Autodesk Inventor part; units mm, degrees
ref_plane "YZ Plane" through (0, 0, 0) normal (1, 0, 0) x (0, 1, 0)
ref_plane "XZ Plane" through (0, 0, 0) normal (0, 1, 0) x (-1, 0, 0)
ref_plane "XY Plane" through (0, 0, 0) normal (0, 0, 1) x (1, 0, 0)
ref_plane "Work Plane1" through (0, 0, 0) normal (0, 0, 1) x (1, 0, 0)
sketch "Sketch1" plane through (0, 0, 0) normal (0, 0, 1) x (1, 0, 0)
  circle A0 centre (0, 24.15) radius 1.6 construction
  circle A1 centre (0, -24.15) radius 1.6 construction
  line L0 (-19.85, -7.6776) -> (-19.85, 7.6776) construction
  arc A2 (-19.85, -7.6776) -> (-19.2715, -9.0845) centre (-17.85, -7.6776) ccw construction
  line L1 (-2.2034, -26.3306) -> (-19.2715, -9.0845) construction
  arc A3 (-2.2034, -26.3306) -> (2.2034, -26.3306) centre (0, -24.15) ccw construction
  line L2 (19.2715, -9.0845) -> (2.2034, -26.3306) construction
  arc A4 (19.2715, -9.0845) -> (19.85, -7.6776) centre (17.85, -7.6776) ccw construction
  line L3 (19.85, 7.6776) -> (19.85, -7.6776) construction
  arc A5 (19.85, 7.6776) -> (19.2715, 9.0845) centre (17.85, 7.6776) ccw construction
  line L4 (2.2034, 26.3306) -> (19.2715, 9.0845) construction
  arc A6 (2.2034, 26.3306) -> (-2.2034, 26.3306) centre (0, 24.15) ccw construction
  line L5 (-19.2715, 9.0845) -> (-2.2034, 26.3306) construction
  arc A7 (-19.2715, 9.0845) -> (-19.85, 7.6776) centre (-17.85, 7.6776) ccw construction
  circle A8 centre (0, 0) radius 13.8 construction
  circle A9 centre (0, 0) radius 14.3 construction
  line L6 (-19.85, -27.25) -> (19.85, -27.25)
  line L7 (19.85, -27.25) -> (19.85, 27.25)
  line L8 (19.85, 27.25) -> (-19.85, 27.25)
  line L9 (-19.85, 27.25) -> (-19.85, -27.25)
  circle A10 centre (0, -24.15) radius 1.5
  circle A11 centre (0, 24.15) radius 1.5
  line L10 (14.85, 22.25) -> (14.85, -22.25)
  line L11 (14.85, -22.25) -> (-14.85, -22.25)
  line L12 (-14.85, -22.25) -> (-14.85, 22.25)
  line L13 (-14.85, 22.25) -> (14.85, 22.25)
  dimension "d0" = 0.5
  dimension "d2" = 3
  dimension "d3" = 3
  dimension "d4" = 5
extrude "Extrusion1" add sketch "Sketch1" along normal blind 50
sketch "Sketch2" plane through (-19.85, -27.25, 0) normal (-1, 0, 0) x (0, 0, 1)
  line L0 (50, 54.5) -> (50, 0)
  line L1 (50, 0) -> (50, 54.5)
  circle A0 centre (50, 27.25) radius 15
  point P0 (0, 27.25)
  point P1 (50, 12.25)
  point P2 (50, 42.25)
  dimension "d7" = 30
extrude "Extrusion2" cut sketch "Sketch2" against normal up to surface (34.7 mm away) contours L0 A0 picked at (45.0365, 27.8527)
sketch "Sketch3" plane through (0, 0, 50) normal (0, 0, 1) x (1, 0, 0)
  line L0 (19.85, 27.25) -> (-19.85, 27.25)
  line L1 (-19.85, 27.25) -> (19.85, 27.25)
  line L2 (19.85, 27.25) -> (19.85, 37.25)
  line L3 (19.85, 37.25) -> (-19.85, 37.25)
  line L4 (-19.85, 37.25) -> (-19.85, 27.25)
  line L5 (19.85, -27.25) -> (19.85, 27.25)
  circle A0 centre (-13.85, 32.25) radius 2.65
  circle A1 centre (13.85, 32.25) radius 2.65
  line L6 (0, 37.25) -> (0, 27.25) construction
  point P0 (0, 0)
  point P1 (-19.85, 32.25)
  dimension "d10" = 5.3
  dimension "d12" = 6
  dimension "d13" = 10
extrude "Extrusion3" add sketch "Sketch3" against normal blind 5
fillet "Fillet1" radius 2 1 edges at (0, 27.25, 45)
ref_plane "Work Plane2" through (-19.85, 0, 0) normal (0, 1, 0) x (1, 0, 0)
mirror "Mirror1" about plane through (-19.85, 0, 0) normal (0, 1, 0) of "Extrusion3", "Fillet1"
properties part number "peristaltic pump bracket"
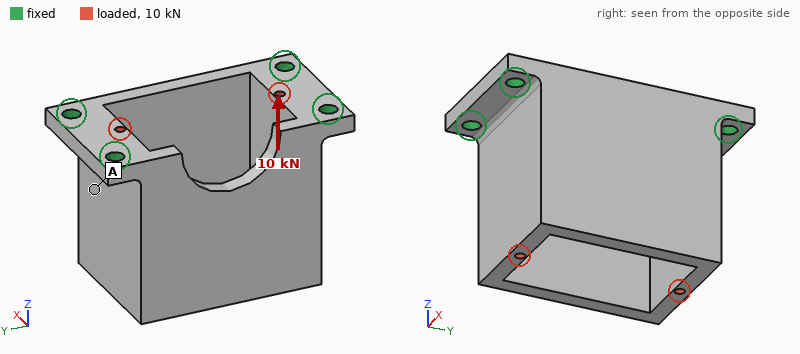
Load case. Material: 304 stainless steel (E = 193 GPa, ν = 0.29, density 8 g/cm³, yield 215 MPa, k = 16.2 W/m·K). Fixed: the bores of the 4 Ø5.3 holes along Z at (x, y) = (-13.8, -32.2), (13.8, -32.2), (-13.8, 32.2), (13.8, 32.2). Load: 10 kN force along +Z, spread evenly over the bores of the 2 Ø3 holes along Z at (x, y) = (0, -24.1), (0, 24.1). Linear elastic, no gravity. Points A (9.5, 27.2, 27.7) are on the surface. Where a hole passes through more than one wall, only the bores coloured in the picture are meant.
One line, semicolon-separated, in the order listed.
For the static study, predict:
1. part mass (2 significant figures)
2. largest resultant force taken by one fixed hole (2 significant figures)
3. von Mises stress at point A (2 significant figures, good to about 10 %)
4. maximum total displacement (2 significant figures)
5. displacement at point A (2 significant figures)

350 g; 2.6 kN; 22 MPa; 9.9 µm; 7.6 µm
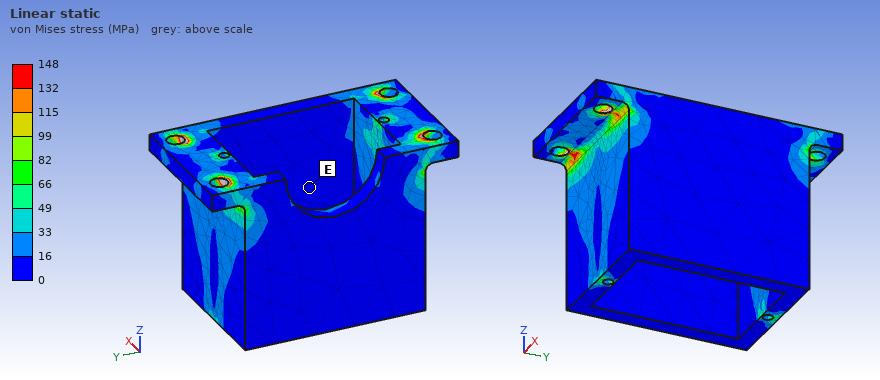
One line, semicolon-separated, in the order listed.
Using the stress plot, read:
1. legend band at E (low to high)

0 to 16 MPa
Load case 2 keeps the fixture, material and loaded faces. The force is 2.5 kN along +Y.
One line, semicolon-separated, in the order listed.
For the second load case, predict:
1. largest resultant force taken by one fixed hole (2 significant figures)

790 N
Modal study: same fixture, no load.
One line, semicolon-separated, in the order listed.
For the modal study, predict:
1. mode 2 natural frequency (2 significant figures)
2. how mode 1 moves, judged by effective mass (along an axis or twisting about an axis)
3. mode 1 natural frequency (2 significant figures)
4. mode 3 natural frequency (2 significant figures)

6500 Hz; along X; 4300 Hz; 6600 Hz
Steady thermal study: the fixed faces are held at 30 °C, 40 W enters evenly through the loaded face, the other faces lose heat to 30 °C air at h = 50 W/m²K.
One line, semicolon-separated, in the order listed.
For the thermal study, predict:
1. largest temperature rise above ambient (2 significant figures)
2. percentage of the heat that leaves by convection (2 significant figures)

64 K; 64 %
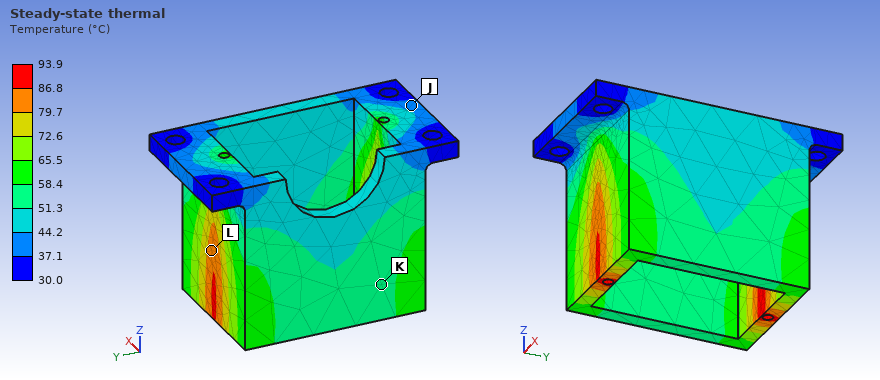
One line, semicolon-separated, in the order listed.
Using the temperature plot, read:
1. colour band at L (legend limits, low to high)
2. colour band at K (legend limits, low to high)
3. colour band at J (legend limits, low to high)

79.7 to 86.8 °C; 51.3 to 58.4 °C; 37.1 to 44.2 °C
